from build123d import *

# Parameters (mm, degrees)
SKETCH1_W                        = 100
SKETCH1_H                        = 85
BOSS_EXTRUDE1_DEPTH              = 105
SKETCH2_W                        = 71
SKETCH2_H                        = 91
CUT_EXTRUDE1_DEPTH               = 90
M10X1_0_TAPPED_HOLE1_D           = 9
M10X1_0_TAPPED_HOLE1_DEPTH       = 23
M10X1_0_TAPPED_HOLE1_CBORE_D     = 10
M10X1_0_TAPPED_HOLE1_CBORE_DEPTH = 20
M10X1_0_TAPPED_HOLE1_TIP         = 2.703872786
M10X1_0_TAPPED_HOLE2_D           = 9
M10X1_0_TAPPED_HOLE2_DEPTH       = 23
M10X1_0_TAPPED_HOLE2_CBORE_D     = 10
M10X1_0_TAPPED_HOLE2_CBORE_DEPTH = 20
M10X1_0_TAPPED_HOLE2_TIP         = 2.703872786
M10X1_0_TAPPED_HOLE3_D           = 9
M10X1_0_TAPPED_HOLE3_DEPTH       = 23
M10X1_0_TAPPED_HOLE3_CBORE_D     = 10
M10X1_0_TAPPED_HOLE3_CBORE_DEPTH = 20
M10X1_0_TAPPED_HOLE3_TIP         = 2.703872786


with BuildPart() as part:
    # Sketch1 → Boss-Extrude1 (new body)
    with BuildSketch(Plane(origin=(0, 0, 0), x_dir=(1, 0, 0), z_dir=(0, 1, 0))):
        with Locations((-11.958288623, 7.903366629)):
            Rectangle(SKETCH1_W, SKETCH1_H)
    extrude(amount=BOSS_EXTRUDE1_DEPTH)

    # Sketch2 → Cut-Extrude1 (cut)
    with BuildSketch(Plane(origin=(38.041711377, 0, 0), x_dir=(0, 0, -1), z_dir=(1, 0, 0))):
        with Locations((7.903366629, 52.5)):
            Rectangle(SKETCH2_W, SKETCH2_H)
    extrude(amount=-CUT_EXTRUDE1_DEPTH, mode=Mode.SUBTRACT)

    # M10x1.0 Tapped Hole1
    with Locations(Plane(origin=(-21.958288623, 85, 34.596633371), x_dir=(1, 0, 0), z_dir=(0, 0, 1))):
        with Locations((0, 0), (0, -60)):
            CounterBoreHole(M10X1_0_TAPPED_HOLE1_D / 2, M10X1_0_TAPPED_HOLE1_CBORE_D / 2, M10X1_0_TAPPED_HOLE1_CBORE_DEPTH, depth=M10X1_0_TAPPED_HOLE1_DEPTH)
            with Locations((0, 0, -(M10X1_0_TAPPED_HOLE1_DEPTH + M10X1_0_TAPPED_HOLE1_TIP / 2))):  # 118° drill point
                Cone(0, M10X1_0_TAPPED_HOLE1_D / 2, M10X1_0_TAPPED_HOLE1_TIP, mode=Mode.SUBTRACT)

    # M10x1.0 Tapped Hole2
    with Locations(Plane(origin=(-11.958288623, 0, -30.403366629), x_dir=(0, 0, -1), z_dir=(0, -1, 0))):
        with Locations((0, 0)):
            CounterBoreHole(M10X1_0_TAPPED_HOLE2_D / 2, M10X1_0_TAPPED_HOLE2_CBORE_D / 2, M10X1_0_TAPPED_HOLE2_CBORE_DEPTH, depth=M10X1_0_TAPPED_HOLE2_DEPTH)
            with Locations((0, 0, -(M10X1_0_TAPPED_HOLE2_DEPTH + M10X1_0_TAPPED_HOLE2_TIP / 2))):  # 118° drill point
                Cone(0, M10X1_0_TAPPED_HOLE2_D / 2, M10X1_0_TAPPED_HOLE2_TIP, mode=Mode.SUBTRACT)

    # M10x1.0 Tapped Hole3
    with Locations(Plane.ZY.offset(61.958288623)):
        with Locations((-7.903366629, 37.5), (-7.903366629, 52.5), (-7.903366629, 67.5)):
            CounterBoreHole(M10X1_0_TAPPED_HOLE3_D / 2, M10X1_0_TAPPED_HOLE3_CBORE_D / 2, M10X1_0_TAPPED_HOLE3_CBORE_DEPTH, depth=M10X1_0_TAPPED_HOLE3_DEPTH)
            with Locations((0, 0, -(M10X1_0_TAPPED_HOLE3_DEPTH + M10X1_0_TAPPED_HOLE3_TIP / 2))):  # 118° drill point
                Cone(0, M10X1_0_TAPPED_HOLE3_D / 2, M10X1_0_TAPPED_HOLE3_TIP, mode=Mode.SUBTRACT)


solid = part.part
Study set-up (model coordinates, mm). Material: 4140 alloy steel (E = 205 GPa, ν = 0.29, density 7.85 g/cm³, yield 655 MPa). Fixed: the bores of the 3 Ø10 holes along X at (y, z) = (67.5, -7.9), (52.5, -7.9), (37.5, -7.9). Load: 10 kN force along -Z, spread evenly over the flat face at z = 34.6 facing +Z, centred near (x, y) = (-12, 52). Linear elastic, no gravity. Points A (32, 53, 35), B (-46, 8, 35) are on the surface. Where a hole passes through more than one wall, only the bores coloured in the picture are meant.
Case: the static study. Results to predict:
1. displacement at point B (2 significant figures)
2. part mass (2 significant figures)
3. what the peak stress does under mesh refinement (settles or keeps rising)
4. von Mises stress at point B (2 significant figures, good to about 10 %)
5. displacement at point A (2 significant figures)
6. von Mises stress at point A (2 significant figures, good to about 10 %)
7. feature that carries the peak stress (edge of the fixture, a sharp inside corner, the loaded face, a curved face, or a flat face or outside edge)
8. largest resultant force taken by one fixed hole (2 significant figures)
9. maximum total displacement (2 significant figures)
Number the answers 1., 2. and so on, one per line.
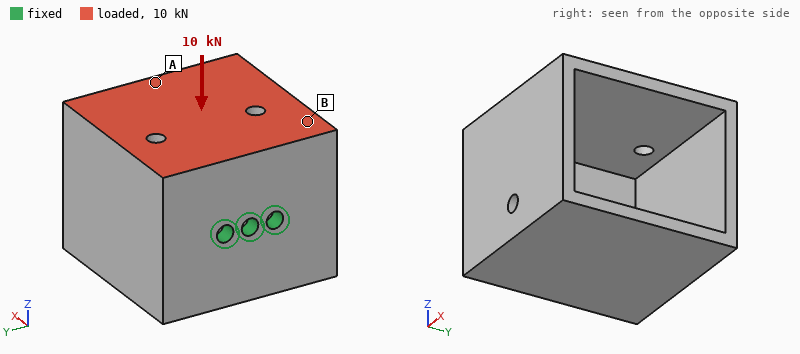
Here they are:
1. 0.093 mm
2. 2.4 kg
3. keeps rising
4. 25 MPa
5. 0.28 mm
6. 72 MPa
7. edge of the fixture
8. 4.5 kN
9. 0.30 mm
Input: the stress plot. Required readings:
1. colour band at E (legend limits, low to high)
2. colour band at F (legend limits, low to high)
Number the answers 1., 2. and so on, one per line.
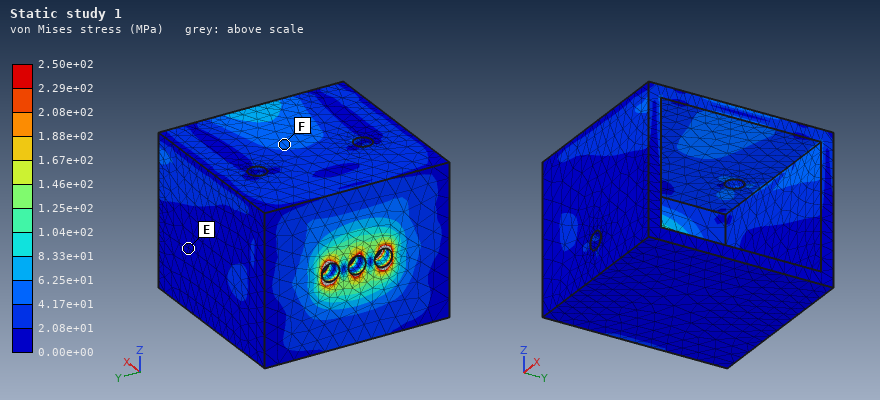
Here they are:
1. 0.00e+00 to 2.08e+01 MPa
2. 4.17e+01 to 6.25e+01 MPa
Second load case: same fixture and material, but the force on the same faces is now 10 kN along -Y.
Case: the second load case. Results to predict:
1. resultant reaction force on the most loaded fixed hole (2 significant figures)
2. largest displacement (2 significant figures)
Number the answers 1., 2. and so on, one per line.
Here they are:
1. 14 kN
2. 0.17 mm
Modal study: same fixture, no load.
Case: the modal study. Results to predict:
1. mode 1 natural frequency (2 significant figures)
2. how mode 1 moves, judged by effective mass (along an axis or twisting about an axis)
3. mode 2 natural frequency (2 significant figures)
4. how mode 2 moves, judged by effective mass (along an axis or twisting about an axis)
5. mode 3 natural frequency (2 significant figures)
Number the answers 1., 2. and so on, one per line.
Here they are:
1. 840 Hz
2. along Z
3. 1100 Hz
4. along Y
5. 1500 Hz
